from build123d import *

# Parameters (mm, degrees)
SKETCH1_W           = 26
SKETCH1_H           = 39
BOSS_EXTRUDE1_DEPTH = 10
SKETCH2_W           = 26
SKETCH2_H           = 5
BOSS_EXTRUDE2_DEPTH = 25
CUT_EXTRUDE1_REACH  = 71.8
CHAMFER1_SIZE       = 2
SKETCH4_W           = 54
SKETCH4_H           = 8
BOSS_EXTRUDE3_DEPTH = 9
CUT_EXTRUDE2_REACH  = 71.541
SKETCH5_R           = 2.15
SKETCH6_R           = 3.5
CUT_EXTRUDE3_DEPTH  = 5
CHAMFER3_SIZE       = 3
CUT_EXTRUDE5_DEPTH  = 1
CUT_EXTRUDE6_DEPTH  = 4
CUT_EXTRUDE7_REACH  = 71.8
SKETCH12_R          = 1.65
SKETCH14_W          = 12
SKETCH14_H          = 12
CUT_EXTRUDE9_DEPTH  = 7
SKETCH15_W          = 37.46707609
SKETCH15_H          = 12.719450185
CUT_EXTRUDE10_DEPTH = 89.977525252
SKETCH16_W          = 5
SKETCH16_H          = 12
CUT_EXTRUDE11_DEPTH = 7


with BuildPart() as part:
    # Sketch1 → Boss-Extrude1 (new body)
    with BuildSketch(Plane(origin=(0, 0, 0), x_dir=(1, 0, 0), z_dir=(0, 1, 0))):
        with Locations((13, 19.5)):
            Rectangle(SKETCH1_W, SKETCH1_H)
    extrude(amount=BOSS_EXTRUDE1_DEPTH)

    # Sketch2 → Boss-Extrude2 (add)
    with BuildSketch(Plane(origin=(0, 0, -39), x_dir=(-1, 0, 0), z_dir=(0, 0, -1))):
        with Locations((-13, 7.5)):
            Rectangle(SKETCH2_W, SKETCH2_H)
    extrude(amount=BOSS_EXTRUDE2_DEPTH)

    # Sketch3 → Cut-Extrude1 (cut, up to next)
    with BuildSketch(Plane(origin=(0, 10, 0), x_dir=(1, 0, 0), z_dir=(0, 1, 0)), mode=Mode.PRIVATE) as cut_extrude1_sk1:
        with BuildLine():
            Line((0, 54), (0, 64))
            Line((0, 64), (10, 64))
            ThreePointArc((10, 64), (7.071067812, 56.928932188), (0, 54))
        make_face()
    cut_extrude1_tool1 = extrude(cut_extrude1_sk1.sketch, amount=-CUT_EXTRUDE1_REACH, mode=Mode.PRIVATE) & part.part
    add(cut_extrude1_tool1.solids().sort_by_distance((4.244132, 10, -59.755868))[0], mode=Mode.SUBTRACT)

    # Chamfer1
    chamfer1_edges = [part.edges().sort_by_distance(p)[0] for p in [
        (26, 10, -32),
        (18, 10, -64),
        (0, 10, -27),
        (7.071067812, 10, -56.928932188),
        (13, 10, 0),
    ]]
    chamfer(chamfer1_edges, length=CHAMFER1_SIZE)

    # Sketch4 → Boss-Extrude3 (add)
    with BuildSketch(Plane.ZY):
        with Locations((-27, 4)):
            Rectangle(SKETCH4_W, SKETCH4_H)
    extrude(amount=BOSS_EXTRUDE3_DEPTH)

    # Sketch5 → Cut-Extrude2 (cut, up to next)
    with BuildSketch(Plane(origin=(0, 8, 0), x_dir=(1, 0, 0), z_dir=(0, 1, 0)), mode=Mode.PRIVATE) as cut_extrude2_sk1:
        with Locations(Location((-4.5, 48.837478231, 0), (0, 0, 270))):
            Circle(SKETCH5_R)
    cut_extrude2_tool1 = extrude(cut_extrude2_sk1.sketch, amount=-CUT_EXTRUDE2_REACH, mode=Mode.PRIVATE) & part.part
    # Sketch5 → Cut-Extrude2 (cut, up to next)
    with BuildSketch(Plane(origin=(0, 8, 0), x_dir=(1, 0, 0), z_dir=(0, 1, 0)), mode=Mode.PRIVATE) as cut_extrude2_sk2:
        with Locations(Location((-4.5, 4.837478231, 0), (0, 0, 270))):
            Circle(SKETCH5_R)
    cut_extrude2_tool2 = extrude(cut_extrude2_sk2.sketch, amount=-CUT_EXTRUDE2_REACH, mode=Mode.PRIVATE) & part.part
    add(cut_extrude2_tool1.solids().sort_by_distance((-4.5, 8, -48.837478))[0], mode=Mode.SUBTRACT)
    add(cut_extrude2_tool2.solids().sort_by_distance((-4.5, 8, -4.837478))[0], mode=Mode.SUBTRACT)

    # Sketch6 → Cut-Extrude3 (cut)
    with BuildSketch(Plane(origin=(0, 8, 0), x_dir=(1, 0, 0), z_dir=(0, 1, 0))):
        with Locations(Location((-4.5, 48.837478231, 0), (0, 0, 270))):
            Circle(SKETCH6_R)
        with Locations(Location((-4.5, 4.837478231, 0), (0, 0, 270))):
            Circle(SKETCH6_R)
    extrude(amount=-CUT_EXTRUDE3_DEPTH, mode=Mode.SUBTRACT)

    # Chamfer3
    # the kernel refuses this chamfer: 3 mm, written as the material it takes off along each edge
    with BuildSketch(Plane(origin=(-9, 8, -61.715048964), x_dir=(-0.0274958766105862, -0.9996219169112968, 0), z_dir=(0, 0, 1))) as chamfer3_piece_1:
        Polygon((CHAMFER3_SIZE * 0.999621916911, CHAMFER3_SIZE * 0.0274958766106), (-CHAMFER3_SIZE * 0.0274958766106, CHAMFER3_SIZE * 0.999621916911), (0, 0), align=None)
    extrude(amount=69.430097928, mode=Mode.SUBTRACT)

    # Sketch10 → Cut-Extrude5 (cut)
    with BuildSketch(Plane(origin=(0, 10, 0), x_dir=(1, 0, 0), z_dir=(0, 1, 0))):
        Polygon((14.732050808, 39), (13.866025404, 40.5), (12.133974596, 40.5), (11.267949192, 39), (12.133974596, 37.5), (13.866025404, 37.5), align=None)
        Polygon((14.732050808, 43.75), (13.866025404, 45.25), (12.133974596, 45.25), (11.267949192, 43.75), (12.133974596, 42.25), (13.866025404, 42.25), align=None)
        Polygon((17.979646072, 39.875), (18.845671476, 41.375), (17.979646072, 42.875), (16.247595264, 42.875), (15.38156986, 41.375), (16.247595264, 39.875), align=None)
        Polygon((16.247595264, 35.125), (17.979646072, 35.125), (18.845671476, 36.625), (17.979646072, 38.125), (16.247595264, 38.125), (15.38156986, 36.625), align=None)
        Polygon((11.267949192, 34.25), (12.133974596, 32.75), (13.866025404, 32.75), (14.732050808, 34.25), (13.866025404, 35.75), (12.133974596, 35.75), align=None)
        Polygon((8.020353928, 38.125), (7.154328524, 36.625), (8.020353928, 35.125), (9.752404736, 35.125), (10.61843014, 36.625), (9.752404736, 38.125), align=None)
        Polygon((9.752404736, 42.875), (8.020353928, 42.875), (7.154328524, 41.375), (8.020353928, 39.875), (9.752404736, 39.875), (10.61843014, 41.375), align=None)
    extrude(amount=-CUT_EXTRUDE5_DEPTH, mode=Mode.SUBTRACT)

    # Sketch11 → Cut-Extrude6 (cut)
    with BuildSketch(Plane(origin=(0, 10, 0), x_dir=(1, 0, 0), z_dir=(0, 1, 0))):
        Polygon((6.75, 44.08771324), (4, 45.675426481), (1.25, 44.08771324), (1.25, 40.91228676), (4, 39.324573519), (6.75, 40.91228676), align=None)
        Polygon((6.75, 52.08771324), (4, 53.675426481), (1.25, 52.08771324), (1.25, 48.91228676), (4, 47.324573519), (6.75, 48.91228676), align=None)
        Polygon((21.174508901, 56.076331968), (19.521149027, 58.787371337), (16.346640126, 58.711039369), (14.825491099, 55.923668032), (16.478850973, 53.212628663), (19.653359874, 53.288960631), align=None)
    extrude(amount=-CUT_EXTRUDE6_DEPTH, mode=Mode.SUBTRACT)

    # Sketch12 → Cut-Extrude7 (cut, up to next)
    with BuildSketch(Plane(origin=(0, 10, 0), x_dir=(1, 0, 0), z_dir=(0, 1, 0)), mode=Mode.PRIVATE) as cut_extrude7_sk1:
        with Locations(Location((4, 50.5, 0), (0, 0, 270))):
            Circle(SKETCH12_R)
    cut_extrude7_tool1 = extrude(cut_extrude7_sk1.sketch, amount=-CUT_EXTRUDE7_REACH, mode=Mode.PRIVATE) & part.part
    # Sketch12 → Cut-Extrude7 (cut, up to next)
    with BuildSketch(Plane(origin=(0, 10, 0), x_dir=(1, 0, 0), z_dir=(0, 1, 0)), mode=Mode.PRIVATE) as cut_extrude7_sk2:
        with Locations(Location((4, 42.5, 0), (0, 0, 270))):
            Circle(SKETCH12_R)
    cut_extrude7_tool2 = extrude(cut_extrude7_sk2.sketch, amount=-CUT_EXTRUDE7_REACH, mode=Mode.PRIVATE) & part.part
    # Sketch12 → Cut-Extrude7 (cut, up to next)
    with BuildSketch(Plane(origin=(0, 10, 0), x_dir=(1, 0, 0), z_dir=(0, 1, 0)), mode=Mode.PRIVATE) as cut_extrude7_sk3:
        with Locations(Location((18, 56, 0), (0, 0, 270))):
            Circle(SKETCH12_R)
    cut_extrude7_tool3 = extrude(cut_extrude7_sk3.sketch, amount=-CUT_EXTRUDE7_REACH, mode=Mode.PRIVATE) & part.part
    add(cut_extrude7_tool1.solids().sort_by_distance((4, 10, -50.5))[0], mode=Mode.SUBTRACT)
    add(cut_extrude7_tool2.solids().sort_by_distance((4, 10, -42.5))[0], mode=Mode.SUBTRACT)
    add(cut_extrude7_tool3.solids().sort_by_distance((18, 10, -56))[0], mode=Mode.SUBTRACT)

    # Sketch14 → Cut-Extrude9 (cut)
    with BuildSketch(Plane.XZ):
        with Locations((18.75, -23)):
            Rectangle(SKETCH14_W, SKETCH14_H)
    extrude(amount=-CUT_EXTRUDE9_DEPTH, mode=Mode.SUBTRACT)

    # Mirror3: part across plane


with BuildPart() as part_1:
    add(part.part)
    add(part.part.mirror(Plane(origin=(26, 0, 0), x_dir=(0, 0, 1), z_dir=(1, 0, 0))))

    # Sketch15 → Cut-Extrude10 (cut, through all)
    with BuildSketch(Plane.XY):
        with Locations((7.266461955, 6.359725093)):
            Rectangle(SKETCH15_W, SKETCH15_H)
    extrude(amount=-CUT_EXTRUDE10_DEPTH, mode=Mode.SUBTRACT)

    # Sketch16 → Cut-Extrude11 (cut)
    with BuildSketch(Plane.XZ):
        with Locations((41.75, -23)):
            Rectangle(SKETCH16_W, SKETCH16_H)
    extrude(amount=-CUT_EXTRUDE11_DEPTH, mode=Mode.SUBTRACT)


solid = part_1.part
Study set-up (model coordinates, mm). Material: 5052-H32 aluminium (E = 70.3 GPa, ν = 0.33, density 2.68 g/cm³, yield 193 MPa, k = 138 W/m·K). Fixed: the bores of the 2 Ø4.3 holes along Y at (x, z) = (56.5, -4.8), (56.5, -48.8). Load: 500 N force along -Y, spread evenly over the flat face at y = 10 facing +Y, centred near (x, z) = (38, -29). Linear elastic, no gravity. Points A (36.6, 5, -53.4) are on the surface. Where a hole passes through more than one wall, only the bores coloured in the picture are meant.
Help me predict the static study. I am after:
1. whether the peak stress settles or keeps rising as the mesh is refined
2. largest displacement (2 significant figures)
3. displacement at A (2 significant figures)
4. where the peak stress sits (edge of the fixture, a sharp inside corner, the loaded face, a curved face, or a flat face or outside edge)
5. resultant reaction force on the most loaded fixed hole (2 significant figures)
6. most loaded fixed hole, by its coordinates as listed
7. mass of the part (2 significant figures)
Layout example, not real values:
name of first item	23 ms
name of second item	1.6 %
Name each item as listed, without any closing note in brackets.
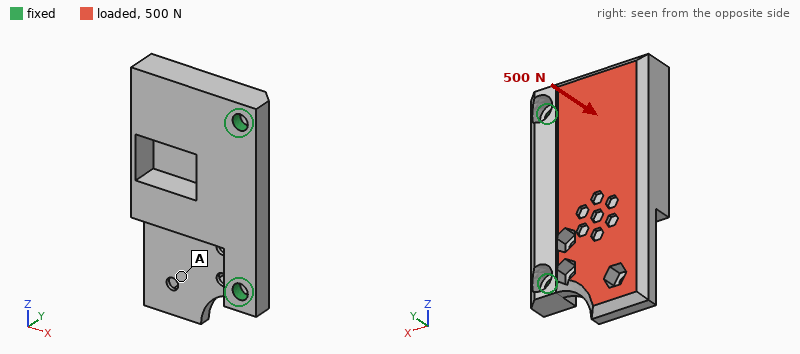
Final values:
whether the peak stress settles or keeps rising as the mesh is refined	keeps rising
largest displacement	0.12 mm
displacement at A	0.072 mm
where the peak stress sits	edge of the fixture
resultant reaction force on the most loaded fixed hole	300 N
most loaded fixed hole, by its coordinates as listed	(56.5, -48.8)
mass of the part	38 g
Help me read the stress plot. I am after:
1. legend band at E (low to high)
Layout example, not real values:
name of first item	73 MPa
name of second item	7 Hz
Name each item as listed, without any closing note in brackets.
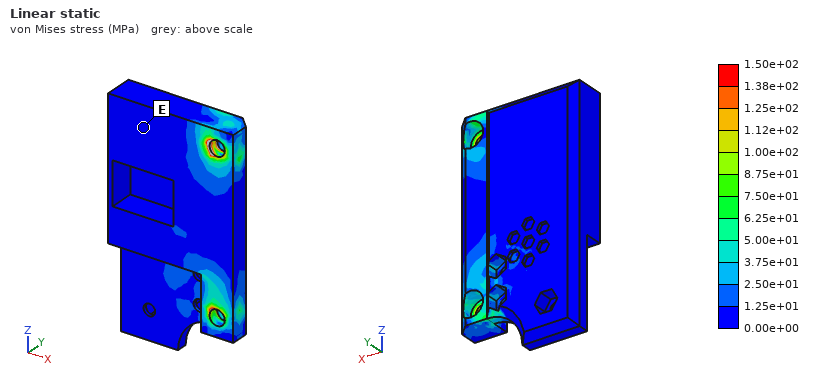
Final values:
legend band at E	0.00e+00 to 1.25e+01 MPa
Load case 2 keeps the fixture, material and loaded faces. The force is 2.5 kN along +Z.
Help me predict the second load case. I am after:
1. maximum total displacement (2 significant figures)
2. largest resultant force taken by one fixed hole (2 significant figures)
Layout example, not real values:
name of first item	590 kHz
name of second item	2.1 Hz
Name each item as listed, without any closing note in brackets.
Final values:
maximum total displacement	62 µm
largest resultant force taken by one fixed hole	1.7 kN
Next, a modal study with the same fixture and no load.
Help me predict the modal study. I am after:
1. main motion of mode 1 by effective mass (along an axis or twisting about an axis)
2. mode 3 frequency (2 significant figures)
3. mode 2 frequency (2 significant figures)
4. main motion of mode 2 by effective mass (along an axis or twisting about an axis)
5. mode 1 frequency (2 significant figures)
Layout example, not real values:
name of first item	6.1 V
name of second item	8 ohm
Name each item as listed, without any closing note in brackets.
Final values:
main motion of mode 1 by effective mass	along Y
mode 3 frequency	9800 Hz
mode 2 frequency	5600 Hz
main motion of mode 2 by effective mass	twisting about X
mode 1 frequency	2500 Hz
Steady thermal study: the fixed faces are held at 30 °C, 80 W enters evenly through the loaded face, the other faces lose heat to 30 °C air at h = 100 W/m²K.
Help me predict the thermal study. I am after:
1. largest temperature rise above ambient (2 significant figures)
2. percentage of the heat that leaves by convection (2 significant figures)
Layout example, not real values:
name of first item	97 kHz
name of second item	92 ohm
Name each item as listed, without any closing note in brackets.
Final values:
largest temperature rise above ambient	54 K
percentage of the heat that leaves by convection	22 %
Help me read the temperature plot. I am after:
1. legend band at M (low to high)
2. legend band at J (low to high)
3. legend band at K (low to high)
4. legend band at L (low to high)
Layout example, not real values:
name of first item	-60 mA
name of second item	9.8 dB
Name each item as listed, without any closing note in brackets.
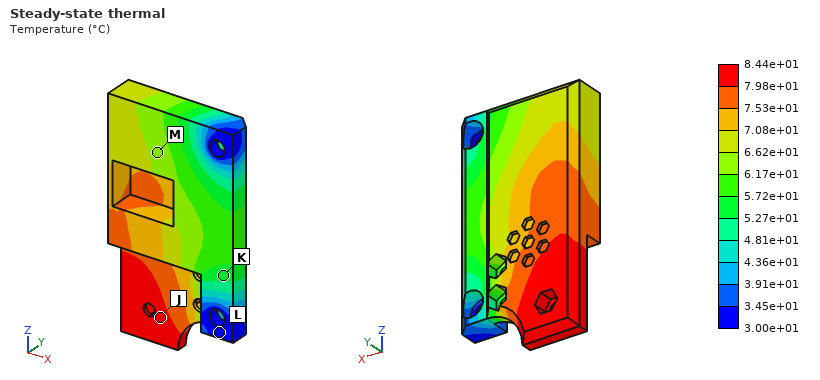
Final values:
legend band at M	6.17e+01 to 6.62e+01 °C
legend band at J	7.98e+01 to 8.44e+01 °C
legend band at K	5.27e+01 to 5.72e+01 °C
legend band at L	3.00e+01 to 3.45e+01 °C
